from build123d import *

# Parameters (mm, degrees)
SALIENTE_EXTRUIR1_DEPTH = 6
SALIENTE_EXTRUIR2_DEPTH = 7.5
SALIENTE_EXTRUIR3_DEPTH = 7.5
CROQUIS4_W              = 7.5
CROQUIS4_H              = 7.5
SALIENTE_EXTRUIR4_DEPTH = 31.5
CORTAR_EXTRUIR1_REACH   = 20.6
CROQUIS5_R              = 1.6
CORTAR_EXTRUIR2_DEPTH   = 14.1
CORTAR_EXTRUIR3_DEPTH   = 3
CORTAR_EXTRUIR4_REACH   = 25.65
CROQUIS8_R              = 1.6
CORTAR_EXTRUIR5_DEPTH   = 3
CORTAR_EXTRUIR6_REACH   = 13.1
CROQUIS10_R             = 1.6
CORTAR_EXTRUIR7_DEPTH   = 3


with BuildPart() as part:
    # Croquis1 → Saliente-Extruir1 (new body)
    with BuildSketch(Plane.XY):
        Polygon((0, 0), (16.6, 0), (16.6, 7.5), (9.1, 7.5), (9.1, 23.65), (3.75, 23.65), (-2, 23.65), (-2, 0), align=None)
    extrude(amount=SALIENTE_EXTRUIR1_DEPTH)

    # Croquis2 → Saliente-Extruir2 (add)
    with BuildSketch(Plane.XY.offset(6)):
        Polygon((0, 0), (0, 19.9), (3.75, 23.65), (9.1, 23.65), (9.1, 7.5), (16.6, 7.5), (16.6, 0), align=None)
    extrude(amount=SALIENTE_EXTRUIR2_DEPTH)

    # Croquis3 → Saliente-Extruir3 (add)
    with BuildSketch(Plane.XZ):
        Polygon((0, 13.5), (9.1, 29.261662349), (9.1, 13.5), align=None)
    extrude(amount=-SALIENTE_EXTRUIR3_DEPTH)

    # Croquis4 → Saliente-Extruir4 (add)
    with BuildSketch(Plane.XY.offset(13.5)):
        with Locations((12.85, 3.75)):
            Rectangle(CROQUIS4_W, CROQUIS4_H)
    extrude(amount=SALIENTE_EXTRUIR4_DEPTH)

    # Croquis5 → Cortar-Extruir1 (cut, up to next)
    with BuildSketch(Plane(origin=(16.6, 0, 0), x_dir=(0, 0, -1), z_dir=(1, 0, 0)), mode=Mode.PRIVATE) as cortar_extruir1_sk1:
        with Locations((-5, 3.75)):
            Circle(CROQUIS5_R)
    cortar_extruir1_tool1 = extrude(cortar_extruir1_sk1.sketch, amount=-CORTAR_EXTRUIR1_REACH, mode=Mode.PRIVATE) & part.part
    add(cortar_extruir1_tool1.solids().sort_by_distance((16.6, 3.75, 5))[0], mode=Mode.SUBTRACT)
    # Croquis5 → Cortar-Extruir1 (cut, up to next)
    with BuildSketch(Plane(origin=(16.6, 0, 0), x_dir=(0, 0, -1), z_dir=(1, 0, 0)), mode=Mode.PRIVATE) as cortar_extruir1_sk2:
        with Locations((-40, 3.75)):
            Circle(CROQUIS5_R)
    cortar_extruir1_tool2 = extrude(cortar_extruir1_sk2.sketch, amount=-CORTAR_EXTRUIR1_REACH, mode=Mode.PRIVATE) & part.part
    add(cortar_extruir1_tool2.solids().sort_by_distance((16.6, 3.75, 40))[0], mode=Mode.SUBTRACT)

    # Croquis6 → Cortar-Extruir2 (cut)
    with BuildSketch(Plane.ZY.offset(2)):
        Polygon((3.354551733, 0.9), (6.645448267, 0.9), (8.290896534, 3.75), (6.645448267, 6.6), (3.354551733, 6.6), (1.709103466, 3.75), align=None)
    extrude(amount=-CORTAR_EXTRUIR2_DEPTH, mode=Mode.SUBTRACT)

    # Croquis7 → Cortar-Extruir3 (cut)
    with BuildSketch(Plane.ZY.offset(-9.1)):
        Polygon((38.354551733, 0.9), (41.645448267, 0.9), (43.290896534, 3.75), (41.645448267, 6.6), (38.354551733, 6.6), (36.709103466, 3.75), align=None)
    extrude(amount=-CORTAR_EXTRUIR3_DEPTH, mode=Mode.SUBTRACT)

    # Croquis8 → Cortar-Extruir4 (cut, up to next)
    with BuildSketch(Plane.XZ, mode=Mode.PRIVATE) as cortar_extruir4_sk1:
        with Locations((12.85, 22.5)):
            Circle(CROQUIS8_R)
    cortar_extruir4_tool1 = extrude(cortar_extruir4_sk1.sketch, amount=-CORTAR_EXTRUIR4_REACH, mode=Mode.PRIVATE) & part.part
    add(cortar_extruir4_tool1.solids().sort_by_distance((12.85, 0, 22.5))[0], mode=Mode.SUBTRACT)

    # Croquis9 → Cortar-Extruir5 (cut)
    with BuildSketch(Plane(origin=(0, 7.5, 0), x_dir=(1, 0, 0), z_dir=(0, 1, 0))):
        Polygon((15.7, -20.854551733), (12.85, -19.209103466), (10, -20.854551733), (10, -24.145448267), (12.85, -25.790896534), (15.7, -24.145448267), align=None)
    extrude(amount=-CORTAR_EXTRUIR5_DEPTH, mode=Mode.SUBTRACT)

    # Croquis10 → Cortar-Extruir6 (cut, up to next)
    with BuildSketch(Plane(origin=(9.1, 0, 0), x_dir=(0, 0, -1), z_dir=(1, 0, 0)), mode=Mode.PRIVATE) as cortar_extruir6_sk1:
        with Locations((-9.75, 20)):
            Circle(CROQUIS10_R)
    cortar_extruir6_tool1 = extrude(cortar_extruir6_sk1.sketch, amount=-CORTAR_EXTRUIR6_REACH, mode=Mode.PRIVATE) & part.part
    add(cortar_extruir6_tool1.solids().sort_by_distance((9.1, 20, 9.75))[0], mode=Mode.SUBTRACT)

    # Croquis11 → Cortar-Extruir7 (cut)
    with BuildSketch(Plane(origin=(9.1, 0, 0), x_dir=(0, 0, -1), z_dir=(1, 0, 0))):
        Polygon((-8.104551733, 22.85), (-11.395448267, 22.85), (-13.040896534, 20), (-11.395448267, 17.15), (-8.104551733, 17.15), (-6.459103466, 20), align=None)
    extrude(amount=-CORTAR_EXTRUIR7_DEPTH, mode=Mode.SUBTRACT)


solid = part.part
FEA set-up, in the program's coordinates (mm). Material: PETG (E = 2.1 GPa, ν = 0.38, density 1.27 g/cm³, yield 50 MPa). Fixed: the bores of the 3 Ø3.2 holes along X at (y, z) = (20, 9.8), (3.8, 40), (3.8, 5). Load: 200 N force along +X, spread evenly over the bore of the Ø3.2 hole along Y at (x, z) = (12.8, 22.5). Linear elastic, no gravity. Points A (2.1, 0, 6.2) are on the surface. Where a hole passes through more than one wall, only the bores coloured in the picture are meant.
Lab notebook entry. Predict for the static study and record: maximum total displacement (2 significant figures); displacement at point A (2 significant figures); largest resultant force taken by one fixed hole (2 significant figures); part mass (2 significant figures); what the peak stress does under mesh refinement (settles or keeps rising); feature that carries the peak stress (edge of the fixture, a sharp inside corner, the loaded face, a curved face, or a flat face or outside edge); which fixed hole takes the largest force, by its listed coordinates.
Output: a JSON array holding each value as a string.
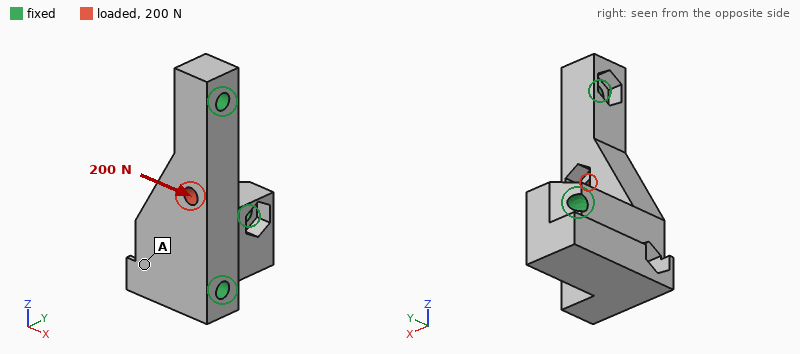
["0.11 mm", "0.041 mm", "130 N", "6.9 g", "keeps rising", "edge of the fixture", "(3.8, 5)"]
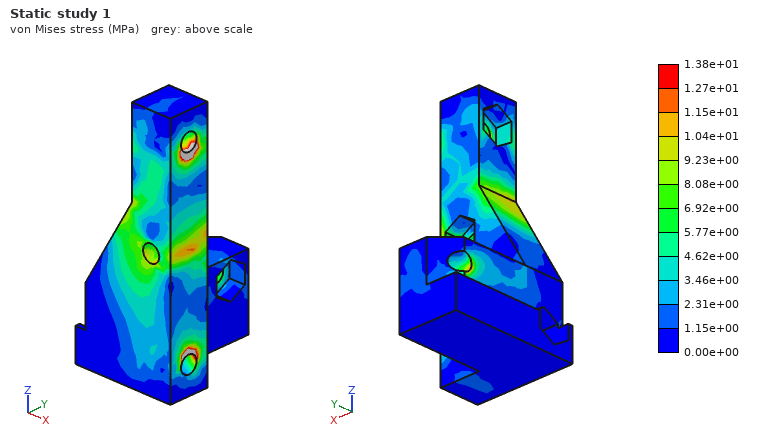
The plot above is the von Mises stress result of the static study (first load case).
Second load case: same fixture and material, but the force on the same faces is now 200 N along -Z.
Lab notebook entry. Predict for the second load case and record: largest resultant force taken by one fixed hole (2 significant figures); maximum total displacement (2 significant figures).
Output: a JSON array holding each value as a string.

["99 N", "23 µm"]
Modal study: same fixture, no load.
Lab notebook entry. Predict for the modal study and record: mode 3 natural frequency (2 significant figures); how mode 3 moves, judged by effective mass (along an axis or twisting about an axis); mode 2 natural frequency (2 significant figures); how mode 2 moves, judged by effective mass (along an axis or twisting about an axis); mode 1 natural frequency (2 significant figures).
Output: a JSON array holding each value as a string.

["8200 Hz", "along X", "6300 Hz", "along Y", "5400 Hz"]
